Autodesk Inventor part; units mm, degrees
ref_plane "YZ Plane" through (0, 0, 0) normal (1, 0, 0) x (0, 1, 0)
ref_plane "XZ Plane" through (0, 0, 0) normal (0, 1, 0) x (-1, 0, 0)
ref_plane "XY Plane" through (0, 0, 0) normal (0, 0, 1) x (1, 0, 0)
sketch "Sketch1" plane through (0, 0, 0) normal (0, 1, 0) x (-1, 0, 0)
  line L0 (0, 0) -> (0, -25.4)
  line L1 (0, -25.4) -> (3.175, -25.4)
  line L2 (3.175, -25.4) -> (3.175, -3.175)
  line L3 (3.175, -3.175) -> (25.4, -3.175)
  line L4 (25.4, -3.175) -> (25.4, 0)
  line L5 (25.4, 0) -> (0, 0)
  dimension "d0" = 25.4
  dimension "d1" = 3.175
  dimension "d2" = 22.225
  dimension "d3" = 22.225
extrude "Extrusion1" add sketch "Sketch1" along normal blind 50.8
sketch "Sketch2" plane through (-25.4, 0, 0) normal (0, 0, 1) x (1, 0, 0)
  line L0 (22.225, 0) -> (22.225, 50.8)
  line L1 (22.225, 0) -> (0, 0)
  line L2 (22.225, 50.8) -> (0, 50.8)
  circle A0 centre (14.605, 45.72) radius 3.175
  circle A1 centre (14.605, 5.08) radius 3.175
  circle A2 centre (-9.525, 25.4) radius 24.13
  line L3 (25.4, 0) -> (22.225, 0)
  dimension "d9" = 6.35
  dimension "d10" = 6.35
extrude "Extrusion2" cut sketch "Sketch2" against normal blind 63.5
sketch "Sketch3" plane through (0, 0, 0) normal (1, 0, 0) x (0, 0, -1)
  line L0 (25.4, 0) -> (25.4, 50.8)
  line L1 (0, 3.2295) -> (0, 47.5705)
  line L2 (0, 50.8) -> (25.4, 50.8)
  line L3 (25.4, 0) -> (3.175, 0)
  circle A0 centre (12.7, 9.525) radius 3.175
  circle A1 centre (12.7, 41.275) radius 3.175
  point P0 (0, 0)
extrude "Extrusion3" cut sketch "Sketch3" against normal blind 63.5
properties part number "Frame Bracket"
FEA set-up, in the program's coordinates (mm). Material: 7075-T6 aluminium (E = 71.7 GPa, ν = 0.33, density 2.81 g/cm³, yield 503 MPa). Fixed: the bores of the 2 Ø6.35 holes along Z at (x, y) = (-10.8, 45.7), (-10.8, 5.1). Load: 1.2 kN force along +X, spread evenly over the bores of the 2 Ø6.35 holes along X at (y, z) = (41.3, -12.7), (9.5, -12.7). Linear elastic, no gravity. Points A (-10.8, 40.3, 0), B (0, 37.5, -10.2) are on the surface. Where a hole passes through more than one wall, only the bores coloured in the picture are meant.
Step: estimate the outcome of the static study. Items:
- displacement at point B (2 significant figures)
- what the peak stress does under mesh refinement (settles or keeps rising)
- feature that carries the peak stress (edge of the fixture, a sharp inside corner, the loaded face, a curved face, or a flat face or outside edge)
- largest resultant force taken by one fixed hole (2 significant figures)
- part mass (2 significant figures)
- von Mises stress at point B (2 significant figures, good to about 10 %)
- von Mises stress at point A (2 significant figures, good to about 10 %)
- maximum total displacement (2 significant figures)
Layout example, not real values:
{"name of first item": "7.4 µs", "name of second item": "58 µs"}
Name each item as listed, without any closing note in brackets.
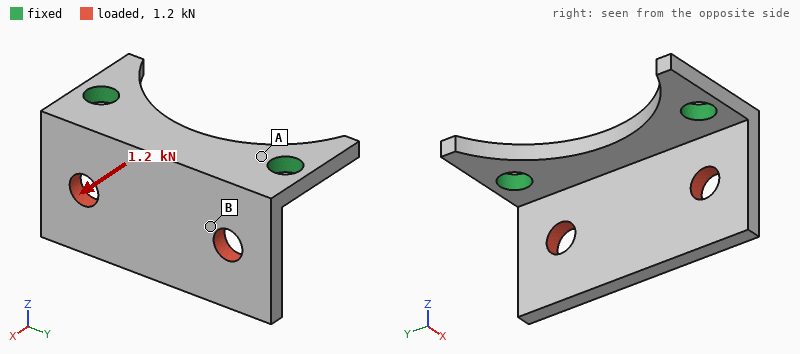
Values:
{"displacement at point B": "0.16 mm", "what the peak stress does under mesh refinement": "keeps rising", "feature that carries the peak stress": "edge of the fixture", "largest resultant force taken by one fixed hole": "630 N", "part mass": "16 g", "von Mises stress at point B": "43 MPa", "von Mises stress at point A": "87 MPa", "maximum total displacement": "0.43 mm"}
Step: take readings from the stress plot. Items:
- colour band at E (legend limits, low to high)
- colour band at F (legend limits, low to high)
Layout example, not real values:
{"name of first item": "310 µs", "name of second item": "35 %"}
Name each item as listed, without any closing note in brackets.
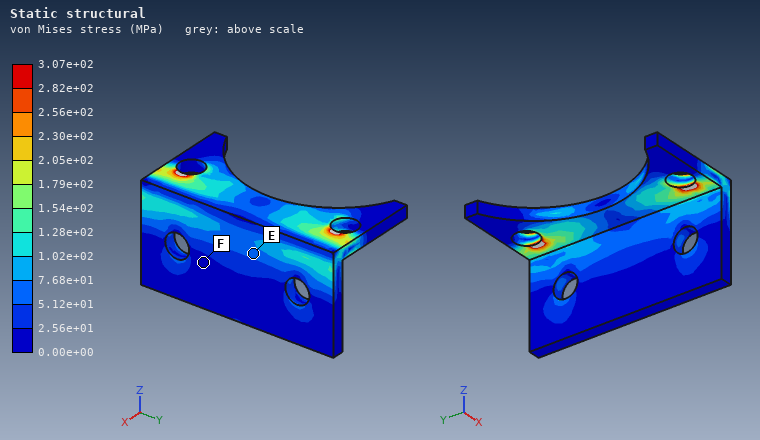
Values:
{"colour band at E": "5.12e+01 to 7.68e+01 MPa", "colour band at F": "0.00e+00 to 2.56e+01 MPa"}
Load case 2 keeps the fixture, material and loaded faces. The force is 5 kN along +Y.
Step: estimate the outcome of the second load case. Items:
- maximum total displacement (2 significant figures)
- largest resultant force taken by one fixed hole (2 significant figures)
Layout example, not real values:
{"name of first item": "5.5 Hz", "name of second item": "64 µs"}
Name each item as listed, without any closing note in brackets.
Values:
{"maximum total displacement": "0.16 mm", "largest resultant force taken by one fixed hole": "3.0 kN"}
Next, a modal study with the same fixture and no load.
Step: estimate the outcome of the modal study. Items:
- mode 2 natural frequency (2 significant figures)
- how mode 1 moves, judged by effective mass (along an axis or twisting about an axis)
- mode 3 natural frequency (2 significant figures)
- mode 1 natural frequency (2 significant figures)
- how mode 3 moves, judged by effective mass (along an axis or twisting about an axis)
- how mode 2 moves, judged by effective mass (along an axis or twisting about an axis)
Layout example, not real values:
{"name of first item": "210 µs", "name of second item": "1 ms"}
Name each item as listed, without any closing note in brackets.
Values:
{"mode 2 natural frequency": "5400 Hz", "how mode 1 moves, judged by effective mass": "along X", "mode 3 natural frequency": "10 kHz", "mode 1 natural frequency": "2900 Hz", "how mode 3 moves, judged by effective mass": "along Z", "how mode 2 moves, judged by effective mass": "twisting about Z"}
